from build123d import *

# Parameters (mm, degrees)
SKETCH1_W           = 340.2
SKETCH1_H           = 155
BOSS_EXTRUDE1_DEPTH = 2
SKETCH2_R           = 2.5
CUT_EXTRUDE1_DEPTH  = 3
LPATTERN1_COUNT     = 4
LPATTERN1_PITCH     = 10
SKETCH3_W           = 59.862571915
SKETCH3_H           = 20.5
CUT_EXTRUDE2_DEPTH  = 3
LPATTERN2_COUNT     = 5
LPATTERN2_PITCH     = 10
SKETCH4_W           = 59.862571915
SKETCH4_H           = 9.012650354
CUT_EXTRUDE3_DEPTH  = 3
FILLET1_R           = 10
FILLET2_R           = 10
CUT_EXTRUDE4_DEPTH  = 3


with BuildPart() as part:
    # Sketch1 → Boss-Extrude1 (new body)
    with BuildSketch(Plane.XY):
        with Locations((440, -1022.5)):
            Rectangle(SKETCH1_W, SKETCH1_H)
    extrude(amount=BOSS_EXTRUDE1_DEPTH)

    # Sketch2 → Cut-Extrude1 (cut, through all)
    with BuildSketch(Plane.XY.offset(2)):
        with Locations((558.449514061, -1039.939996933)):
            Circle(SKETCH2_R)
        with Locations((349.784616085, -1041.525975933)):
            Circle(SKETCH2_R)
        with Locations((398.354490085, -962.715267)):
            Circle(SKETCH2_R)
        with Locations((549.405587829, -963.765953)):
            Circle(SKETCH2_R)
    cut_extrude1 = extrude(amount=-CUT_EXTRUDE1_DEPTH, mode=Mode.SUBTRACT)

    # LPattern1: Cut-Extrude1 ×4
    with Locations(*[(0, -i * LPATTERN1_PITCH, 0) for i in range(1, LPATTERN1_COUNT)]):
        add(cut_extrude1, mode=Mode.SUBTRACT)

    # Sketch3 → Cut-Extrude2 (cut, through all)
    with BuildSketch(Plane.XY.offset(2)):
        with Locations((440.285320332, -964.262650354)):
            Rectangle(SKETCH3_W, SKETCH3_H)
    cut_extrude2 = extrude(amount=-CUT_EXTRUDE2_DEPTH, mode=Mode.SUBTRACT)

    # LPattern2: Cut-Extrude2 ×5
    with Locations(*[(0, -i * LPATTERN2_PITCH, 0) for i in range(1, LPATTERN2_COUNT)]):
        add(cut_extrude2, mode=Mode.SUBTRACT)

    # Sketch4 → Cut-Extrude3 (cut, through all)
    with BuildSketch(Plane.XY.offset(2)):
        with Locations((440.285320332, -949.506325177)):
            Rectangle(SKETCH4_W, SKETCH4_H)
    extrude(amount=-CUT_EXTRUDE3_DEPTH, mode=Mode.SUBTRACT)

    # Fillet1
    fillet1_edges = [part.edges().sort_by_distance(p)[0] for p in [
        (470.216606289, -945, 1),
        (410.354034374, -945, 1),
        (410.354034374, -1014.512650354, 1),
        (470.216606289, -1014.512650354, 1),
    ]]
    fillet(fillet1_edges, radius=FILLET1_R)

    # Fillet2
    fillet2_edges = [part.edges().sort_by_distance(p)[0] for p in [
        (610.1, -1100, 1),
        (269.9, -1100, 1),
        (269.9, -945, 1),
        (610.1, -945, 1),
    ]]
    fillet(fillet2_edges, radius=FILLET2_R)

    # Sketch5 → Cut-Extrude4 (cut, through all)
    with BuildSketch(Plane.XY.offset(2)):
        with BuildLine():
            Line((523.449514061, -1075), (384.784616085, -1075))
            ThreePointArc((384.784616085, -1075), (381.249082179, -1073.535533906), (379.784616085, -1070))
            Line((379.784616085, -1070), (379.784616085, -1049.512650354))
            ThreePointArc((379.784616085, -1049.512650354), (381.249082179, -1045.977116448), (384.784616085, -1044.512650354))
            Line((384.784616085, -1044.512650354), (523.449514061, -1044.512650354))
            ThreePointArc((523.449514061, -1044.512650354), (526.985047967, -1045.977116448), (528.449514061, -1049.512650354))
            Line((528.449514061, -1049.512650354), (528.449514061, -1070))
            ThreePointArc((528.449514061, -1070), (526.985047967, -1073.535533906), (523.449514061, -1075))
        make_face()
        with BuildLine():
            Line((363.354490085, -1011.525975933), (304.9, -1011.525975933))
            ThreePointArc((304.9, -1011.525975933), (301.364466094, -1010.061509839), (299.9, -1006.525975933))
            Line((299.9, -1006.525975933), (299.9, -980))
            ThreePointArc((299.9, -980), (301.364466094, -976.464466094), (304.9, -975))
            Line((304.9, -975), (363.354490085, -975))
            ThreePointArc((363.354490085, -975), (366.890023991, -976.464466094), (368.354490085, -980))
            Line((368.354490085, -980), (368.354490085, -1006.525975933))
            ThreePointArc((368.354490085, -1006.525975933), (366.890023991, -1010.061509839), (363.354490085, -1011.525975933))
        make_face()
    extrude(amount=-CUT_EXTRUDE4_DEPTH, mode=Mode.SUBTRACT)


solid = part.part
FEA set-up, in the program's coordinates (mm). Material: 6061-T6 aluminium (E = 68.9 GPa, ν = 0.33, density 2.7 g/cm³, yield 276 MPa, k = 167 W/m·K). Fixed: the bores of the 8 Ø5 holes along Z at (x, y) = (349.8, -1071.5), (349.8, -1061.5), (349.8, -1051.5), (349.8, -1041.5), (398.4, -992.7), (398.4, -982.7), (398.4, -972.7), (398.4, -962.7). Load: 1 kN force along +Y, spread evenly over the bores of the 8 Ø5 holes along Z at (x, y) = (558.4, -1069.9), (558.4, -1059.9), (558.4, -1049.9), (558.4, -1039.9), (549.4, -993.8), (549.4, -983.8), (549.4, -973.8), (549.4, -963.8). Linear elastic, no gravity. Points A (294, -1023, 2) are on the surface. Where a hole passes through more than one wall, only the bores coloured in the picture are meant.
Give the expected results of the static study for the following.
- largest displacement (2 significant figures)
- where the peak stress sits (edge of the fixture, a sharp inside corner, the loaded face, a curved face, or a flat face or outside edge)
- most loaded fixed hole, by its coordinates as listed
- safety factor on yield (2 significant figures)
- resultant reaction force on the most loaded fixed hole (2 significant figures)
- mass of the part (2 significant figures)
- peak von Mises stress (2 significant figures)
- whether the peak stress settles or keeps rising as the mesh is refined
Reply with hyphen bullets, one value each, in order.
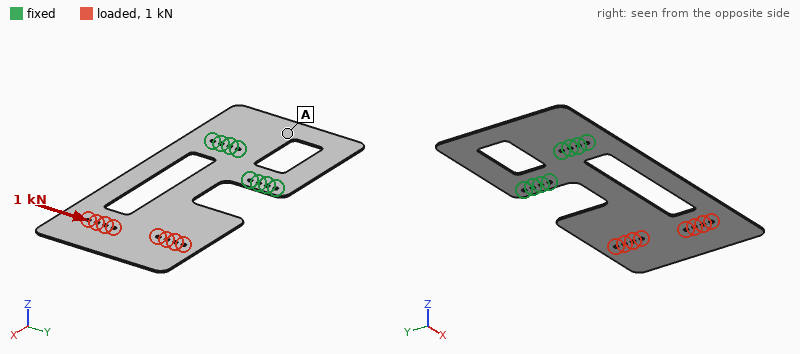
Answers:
- 0.93 mm
- a curved face
- (349.8, -1071.5)
- 1.1
- 1.8 kN
- 220 g
- 260 MPa
- settles
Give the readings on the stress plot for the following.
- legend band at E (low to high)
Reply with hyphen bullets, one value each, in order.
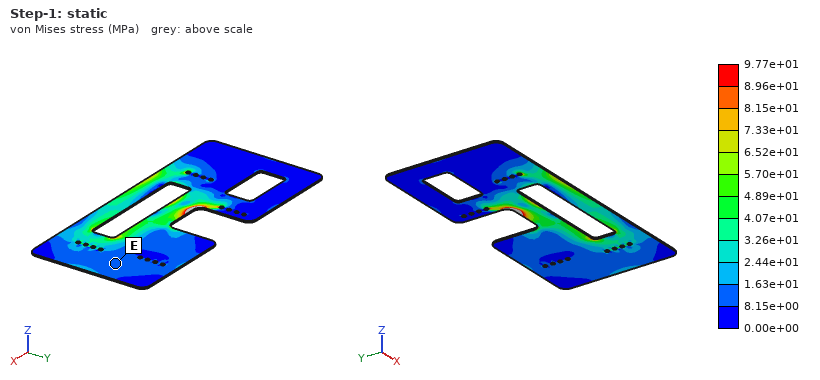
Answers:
- 8.15e+00 to 1.63e+01 MPa
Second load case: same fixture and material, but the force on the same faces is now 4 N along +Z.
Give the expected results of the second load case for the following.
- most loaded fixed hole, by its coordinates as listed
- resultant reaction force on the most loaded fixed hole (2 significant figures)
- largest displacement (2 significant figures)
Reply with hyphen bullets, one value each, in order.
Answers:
- (398.4, -992.7)
- 16 N
- 3.9 mm
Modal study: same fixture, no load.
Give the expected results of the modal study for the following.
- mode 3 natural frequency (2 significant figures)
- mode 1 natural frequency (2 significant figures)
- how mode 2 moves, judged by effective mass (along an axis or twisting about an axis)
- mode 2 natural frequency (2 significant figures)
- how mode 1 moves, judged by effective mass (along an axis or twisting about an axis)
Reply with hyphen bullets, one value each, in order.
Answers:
- 150 Hz
- 20 Hz
- twisting about X
- 61 Hz
- along Z
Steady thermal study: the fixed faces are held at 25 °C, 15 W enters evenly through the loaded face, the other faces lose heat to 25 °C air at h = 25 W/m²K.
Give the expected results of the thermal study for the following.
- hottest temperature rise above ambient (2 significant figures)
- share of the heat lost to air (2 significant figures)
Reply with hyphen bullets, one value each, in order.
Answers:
- 19 K
- 94 %
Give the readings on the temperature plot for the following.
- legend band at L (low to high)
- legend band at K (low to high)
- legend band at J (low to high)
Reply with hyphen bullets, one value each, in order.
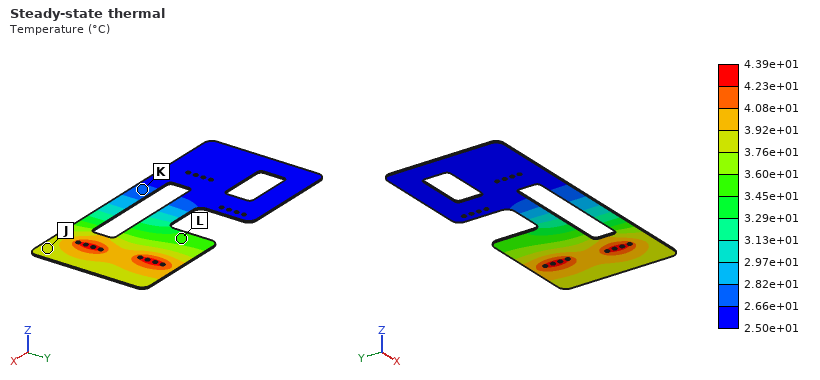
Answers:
- 3.45e+01 to 3.60e+01 °C
- 2.66e+01 to 2.82e+01 °C
- 3.76e+01 to 3.92e+01 °C
